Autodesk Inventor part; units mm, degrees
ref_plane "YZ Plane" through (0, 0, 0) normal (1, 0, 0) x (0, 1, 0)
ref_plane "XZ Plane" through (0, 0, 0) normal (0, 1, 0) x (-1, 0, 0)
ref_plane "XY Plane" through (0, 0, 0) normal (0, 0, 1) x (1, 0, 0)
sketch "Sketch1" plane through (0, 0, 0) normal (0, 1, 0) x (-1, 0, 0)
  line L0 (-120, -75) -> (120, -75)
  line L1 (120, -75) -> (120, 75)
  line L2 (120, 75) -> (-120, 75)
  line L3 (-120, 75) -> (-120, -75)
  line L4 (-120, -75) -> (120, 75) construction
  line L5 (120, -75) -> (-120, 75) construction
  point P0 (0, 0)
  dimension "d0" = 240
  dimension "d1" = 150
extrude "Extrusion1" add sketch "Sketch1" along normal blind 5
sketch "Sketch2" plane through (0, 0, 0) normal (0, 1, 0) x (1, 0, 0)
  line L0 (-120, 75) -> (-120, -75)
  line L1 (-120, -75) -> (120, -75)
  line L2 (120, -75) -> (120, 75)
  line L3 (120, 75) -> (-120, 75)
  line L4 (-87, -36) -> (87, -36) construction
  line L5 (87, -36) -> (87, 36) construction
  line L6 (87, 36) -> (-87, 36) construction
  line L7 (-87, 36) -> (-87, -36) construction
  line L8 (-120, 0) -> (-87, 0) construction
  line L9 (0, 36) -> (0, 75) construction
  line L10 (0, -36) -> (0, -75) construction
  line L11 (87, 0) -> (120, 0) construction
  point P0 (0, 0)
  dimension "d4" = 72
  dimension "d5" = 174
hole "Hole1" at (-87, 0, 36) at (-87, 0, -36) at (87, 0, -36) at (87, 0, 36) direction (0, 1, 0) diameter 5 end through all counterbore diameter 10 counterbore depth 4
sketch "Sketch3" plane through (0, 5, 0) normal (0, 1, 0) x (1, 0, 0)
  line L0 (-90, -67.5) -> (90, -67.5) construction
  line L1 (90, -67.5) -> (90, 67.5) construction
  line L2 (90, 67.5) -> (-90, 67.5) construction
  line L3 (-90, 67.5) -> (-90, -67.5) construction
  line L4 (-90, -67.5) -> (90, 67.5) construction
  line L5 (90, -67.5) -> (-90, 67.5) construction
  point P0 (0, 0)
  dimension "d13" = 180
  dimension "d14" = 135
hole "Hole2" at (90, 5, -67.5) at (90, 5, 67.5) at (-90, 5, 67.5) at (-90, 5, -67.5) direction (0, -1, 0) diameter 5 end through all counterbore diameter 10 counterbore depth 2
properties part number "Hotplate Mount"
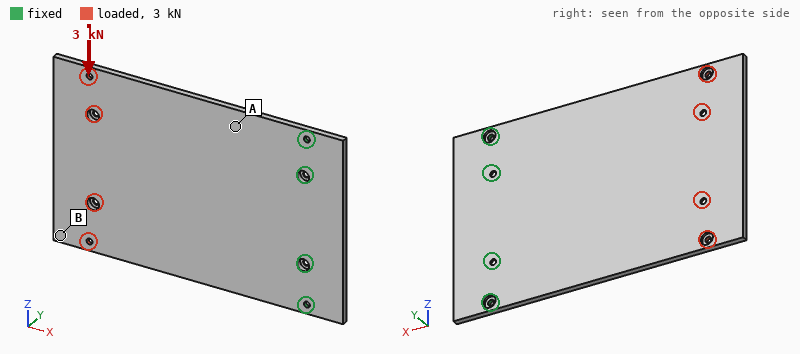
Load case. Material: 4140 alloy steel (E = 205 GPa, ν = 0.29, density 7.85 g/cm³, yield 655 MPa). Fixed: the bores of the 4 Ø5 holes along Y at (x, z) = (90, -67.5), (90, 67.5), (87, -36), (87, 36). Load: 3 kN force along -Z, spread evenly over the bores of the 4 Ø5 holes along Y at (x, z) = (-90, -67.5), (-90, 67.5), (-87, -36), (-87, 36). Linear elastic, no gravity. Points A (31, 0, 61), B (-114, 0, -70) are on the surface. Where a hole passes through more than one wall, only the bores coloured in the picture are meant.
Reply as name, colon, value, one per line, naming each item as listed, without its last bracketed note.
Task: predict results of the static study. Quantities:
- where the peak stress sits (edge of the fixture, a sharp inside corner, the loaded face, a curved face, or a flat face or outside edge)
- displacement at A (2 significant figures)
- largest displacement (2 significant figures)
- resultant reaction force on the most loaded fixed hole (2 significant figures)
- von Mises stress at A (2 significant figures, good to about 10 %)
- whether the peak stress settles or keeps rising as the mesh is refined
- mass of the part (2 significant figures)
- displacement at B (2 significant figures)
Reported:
where the peak stress sits: edge of the fixture
displacement at A: 14 µm
largest displacement: 53 µm
resultant reaction force on the most loaded fixed hole: 3.4 kN
von Mises stress at A: 16 MPa
whether the peak stress settles or keeps rising as the mesh is refined: keeps rising
mass of the part: 1.4 kg
displacement at B: 50 µm
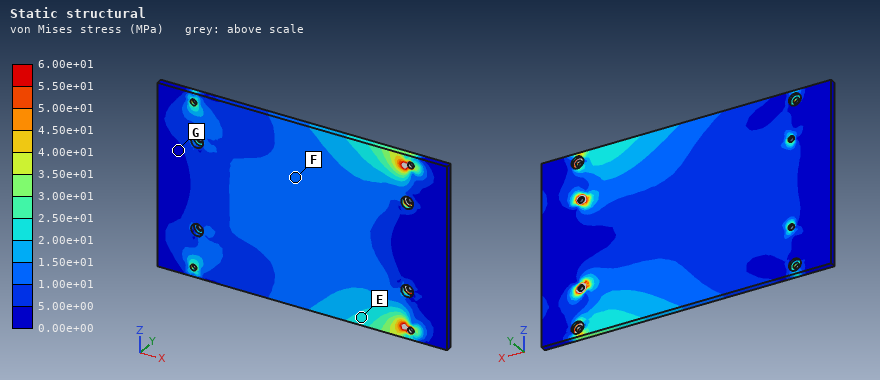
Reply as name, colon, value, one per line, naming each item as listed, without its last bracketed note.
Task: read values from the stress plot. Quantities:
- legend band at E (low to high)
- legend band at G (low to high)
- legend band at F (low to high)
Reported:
legend band at E: 2.00e+01 to 2.50e+01 MPa
legend band at G: 0.00e+00 to 5.00e+00 MPa
legend band at F: 1.00e+01 to 1.50e+01 MPa
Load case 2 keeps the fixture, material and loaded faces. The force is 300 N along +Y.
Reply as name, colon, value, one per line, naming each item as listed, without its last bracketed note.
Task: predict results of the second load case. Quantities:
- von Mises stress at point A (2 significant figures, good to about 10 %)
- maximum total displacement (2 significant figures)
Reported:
von Mises stress at point A: 61 MPa
maximum total displacement: 2.8 mm
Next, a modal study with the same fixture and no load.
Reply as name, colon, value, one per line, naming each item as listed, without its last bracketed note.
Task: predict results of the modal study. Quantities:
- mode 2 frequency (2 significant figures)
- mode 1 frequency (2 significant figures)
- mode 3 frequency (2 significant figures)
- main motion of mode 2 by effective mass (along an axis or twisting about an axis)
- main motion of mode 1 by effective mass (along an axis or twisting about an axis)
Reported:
mode 2 frequency: 300 Hz
mode 1 frequency: 83 Hz
mode 3 frequency: 540 Hz
main motion of mode 2 by effective mass: twisting about X
main motion of mode 1 by effective mass: along Y
